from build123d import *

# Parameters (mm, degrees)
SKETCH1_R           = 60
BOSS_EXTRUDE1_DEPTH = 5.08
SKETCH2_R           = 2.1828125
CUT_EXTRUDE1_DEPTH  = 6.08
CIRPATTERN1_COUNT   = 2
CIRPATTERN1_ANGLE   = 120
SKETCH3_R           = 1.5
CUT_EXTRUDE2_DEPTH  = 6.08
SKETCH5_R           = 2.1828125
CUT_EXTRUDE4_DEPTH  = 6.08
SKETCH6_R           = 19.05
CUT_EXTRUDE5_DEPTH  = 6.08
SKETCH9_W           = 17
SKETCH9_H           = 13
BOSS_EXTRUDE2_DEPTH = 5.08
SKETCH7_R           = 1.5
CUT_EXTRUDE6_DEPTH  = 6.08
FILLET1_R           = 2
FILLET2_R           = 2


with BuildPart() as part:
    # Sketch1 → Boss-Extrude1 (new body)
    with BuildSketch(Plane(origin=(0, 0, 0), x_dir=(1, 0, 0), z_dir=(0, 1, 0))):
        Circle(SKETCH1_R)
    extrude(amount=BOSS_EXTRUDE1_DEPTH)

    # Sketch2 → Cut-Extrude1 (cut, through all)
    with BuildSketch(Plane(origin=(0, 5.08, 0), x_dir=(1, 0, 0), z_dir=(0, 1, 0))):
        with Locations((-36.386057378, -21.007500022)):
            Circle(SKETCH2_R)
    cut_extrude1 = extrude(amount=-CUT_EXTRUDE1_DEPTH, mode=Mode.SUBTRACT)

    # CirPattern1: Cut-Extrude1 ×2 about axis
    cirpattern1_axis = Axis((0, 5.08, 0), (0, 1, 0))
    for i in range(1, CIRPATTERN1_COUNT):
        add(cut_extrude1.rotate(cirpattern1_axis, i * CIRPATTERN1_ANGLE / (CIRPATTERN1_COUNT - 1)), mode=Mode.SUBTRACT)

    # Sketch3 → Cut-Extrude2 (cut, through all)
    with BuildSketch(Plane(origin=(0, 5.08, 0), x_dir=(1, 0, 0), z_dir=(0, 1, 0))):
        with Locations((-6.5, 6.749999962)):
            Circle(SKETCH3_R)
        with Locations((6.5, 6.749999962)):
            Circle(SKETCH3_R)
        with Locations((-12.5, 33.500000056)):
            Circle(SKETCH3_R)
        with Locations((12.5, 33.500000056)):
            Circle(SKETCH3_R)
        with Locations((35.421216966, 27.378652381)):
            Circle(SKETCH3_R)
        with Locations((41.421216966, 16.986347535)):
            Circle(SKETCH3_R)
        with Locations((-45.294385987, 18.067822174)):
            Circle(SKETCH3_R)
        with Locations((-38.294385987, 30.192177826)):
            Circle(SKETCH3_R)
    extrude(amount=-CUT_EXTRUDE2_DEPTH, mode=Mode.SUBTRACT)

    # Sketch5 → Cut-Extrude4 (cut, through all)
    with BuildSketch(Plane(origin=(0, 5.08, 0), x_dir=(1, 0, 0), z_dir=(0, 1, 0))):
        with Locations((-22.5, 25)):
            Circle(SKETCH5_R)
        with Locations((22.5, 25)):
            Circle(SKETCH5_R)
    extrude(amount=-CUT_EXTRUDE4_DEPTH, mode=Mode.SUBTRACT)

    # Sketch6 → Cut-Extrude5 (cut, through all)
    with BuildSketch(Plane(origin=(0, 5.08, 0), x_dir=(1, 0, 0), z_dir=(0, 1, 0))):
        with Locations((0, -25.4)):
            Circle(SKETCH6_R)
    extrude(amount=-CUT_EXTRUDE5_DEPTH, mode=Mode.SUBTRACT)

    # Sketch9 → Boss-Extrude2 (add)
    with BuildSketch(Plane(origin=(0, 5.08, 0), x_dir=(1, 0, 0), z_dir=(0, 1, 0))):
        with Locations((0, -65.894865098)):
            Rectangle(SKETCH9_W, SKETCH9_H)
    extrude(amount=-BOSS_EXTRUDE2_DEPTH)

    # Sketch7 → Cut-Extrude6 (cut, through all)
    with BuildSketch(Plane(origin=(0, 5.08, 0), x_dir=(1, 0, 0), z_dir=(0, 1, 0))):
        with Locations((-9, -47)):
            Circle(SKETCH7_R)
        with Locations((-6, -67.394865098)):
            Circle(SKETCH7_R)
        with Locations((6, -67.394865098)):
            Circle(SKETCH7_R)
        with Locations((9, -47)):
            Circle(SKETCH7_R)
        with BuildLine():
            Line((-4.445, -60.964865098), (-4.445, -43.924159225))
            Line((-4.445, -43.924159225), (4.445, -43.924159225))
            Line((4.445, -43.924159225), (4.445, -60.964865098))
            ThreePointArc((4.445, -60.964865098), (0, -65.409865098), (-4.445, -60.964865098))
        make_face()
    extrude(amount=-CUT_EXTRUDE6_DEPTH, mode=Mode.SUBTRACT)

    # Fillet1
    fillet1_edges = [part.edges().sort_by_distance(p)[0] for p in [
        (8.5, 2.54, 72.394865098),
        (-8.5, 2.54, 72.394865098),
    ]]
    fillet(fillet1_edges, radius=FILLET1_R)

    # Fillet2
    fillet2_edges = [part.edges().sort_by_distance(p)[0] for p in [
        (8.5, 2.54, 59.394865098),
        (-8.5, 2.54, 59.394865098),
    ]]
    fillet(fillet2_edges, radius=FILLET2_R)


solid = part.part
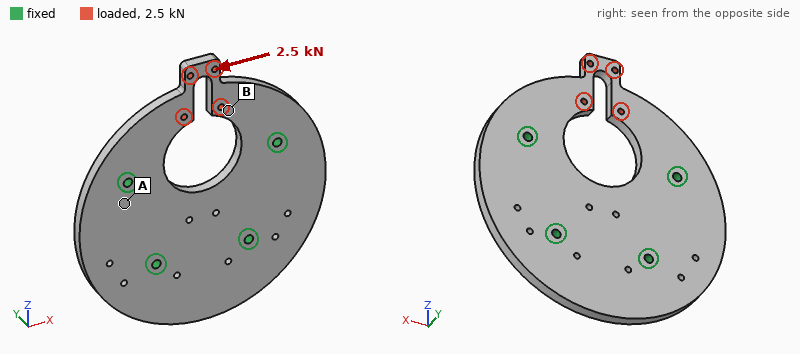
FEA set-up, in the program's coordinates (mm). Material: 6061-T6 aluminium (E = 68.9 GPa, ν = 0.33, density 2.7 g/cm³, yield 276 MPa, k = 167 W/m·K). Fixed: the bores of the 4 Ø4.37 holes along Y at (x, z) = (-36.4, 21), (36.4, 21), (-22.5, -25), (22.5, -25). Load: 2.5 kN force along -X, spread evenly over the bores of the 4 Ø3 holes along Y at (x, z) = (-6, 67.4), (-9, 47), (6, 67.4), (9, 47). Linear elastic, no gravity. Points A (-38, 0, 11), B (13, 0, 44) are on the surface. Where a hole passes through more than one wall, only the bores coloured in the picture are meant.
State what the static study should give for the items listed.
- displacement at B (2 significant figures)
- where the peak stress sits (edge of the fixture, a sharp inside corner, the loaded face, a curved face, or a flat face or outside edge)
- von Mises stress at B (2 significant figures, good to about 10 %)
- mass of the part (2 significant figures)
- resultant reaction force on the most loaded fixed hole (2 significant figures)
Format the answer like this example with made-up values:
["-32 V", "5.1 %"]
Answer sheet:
["23 µm", "a curved face", "14 MPa", "140 g", "1.7 kN"]
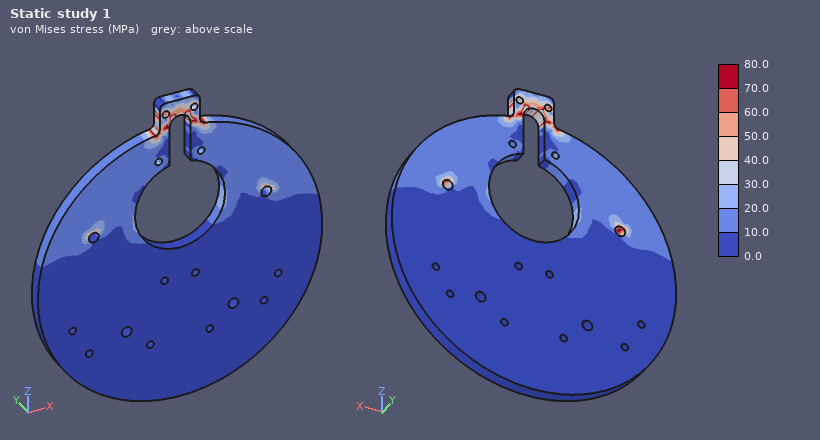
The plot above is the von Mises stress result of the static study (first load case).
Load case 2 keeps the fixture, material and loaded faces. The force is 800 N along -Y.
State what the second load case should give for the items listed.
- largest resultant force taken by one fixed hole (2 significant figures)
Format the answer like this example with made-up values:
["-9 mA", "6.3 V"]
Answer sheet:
["490 N"]
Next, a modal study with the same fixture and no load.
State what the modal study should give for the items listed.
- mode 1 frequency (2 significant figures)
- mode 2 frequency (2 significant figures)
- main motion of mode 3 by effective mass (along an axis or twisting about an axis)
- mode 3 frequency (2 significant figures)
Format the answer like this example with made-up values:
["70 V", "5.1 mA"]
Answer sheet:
["1900 Hz", "3700 Hz", "along Y", "4300 Hz"]
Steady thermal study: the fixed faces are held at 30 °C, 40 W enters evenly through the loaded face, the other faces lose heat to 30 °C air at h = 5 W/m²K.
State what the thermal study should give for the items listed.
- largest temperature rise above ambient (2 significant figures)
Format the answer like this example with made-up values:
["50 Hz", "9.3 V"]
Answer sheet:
["77 K"]
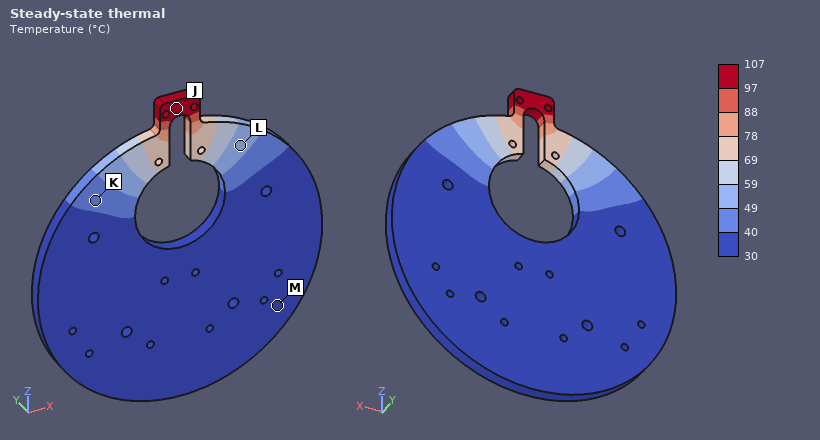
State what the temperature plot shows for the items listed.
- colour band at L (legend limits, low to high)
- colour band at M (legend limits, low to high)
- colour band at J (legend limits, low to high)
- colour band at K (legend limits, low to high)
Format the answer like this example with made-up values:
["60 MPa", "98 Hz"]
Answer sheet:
["49 to 59 °C", "30 to 40 °C", "97 to 107 °C", "40 to 49 °C"]
